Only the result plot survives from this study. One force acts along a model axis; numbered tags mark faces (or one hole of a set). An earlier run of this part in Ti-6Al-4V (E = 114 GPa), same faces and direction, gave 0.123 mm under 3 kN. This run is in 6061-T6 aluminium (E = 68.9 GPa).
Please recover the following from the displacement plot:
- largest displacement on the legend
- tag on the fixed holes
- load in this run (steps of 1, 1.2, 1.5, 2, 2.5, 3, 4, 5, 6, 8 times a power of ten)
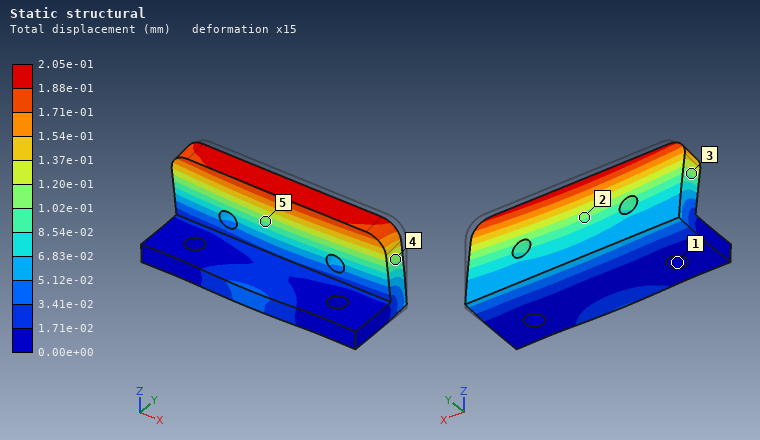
2.05e-01 mm
1
3 kN
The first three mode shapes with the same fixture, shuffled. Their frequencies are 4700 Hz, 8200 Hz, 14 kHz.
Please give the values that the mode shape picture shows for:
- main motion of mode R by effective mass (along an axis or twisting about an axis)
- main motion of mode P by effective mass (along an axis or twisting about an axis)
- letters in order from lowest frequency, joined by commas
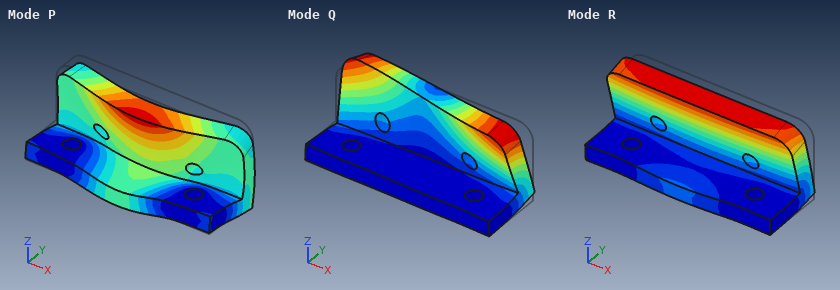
along Y
along Z
R, Q, P
